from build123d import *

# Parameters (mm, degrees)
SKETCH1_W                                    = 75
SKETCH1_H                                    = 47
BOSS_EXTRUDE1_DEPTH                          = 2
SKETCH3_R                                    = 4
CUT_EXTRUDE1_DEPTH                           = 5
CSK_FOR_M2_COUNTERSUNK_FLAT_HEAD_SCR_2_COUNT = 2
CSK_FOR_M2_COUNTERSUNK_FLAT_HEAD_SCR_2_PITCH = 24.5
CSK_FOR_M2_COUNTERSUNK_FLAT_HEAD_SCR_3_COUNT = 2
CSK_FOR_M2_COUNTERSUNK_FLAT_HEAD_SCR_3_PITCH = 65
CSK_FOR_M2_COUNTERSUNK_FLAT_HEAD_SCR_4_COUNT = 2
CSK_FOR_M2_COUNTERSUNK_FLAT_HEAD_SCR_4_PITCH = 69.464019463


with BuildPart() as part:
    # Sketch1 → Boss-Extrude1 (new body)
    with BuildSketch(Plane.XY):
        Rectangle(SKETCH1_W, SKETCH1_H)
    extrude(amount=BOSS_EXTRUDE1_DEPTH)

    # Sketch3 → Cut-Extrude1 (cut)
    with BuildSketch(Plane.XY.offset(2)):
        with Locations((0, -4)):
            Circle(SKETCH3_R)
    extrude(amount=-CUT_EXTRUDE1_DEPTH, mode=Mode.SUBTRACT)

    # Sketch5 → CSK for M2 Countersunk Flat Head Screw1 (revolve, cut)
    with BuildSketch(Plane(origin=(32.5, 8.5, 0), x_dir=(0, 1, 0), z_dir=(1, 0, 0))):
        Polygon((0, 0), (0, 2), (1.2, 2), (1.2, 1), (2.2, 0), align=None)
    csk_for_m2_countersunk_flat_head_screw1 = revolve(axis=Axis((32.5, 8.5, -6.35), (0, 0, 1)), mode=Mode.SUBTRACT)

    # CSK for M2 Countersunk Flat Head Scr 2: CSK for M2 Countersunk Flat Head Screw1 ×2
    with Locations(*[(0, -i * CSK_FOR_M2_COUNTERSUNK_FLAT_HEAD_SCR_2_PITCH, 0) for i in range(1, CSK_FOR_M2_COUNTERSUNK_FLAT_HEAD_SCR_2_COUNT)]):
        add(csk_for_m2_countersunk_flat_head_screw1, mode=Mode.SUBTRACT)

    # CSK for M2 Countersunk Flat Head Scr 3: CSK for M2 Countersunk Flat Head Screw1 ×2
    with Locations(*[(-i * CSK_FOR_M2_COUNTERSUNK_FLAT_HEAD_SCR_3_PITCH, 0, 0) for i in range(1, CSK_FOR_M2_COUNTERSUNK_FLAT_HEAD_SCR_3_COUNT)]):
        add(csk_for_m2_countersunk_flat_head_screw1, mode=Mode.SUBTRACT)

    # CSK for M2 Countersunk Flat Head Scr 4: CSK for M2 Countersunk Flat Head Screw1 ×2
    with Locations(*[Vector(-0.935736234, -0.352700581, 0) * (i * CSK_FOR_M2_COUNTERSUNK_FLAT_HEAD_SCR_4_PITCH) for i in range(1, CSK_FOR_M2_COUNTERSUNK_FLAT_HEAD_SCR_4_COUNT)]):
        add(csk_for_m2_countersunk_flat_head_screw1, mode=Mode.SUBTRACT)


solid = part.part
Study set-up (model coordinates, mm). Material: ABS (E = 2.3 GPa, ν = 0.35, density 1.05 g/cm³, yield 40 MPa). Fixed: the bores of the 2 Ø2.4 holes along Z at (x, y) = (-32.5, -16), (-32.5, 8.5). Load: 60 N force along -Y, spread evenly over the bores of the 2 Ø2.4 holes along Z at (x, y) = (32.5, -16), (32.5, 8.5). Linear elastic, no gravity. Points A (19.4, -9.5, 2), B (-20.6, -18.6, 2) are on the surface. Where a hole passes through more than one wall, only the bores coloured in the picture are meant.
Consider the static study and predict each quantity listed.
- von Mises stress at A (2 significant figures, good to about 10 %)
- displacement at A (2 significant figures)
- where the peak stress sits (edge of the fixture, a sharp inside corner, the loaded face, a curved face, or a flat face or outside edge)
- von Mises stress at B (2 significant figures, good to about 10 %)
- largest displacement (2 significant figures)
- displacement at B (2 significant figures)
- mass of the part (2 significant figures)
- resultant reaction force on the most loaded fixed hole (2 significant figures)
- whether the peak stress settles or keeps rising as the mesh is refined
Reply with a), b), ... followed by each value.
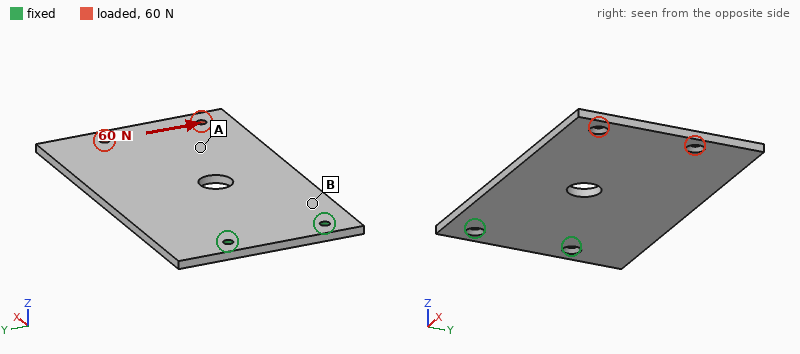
a) 2.4 MPa
b) 0.33 mm
c) edge of the fixture
d) 5.0 MPa
e) 0.79 mm
f) 0.12 mm
g) 7.2 g
h) 160 N
i) keeps rising
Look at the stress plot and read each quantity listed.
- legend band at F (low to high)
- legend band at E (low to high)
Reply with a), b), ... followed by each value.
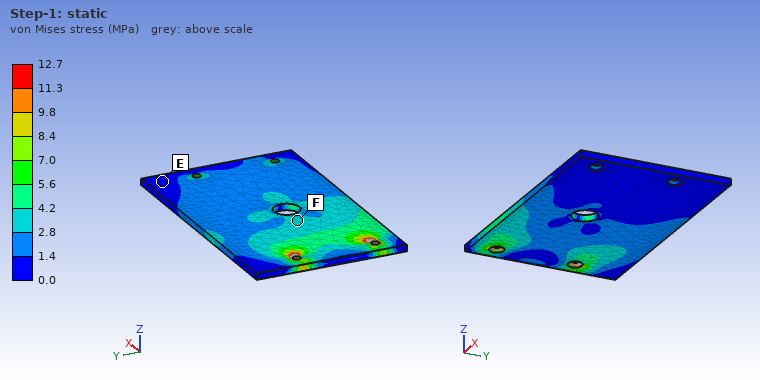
a) 2.8 to 4.2 MPa
b) 0.0 to 1.4 MPa
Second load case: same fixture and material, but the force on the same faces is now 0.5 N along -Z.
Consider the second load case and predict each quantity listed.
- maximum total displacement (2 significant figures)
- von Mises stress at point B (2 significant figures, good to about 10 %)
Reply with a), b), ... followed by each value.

a) 0.90 mm
b) 0.88 MPa
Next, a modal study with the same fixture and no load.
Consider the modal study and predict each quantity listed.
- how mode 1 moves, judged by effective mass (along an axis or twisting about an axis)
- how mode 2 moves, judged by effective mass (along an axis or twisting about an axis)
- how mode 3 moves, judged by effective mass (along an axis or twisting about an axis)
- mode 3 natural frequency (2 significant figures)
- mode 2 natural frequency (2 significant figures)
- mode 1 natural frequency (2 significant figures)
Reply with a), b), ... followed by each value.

a) along Z
b) twisting about X
c) along Z
d) 540 Hz
e) 300 Hz
f) 86 Hz
